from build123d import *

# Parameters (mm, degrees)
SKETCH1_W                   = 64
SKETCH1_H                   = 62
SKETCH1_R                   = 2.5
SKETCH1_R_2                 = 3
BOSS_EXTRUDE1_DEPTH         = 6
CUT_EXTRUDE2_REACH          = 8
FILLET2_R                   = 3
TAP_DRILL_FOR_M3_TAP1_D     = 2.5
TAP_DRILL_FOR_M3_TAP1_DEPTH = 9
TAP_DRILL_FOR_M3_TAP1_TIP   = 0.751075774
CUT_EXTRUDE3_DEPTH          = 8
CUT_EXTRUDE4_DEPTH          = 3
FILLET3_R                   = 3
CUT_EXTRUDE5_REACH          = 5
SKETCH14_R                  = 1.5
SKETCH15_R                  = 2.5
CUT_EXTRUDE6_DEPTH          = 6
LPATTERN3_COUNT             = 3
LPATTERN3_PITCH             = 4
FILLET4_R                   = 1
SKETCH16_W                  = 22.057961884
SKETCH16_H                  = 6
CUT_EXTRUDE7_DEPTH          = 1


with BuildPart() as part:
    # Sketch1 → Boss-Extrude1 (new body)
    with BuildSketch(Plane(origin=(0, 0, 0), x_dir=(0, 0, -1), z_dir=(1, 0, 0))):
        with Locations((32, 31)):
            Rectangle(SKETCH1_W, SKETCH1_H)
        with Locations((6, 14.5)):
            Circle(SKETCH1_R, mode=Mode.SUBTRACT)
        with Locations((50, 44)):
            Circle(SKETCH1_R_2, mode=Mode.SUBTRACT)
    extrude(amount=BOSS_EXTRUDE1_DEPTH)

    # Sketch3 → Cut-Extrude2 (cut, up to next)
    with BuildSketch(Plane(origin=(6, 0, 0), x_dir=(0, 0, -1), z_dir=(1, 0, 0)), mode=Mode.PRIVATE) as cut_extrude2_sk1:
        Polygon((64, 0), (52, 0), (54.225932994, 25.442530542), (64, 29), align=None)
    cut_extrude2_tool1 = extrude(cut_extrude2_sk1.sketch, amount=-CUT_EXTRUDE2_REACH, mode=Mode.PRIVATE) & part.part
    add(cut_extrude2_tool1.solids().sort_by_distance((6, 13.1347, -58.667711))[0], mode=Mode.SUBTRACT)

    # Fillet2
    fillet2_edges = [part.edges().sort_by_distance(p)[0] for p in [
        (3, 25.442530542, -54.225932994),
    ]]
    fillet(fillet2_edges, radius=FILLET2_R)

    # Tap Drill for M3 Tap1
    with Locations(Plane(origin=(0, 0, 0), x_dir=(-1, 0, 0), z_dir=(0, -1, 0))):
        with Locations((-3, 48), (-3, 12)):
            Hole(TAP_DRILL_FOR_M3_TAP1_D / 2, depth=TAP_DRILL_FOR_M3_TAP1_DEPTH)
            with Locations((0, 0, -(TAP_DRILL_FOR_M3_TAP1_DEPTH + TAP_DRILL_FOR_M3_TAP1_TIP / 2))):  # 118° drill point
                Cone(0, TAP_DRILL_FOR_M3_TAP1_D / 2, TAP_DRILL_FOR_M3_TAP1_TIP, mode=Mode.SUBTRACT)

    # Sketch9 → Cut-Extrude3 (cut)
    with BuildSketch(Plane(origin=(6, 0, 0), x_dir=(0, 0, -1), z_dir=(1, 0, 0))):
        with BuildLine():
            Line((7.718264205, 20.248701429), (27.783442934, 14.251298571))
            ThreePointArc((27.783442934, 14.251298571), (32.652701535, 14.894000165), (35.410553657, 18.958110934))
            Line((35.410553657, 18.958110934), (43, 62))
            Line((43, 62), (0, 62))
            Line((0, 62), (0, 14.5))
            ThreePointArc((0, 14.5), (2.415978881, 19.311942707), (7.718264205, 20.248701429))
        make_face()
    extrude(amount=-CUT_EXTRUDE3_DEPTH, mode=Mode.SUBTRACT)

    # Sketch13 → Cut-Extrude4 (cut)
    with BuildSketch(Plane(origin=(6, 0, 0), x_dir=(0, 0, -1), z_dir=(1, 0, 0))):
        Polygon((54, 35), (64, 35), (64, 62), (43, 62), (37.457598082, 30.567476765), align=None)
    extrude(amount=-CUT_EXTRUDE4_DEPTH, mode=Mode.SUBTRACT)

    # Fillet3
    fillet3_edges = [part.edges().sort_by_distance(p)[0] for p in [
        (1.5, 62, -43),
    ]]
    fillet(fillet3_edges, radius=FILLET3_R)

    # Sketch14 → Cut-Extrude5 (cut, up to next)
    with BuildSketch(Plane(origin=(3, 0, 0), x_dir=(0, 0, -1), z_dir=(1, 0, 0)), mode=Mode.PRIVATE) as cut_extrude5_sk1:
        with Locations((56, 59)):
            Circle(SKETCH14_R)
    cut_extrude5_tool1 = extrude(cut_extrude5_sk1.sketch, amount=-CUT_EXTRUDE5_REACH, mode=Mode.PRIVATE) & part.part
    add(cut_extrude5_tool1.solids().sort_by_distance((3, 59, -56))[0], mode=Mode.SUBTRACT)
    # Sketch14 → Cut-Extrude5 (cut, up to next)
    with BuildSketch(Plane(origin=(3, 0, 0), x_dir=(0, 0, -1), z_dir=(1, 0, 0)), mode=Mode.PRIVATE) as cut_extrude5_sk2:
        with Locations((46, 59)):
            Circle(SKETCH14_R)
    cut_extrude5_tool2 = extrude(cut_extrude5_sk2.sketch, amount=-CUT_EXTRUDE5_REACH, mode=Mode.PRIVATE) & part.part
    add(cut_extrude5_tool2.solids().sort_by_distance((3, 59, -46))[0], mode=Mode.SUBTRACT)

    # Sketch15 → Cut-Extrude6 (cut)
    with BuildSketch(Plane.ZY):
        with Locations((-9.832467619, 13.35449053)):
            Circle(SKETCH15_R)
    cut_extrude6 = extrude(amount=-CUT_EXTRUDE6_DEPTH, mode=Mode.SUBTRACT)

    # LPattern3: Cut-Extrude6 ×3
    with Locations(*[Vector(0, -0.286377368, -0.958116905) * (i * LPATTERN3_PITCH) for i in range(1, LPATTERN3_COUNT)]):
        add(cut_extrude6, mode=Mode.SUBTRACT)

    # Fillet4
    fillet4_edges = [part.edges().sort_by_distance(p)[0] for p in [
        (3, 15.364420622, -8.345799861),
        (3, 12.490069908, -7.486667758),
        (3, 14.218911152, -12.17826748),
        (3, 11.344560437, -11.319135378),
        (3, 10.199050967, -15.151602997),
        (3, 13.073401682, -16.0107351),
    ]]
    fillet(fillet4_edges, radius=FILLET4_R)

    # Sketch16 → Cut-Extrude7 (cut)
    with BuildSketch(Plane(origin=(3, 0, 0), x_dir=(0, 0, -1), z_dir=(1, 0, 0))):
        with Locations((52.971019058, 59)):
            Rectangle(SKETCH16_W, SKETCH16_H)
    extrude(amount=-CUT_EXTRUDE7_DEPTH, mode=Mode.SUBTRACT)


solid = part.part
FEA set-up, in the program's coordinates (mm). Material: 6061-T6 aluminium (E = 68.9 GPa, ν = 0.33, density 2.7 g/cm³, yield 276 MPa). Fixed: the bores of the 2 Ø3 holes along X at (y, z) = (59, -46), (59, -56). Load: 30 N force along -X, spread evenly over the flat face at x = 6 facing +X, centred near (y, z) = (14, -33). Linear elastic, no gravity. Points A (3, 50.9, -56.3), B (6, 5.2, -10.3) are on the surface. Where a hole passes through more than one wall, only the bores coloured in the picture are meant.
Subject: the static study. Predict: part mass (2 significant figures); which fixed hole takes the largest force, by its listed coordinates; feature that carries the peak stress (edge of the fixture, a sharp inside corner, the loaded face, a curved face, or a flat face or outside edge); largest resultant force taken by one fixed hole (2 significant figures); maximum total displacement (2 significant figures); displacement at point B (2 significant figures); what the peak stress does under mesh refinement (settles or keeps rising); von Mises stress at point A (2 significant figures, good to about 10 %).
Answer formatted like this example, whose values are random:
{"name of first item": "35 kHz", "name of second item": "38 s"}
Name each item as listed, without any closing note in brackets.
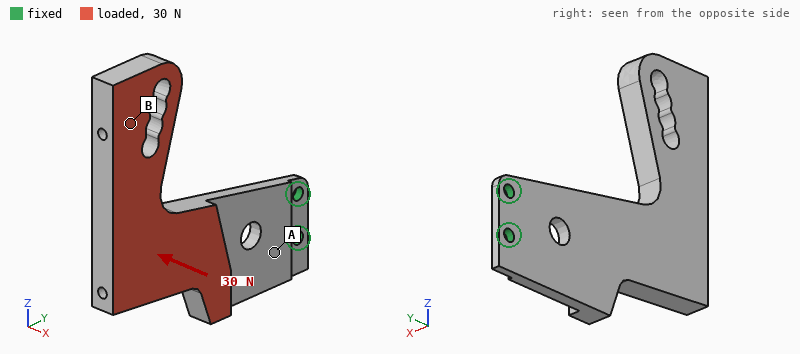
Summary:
{"part mass": "24 g", "which fixed hole takes the largest force, by its listed coordinates": "(59, -46)", "feature that carries the peak stress": "edge of the fixture", "largest resultant force taken by one fixed hole": "50 N", "maximum total displacement": "0.66 mm", "displacement at point B": "0.58 mm", "what the peak stress does under mesh refinement": "keeps rising", "von Mises stress at point A": "32 MPa"}
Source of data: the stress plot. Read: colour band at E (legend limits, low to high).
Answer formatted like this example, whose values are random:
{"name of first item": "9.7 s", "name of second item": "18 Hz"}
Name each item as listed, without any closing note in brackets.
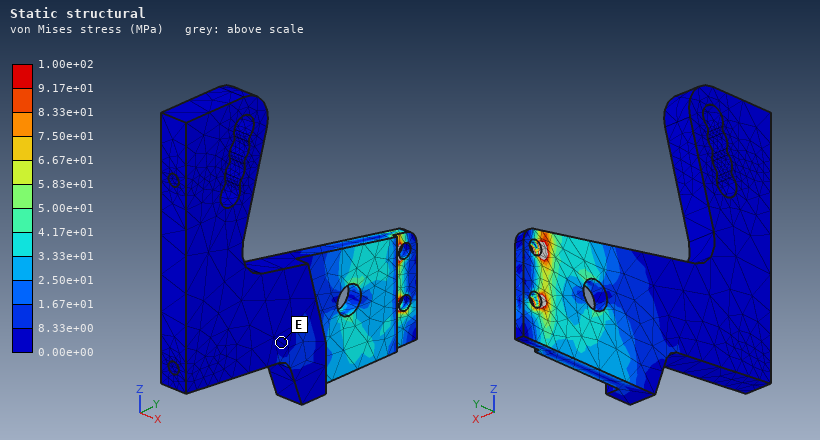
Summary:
{"colour band at E": "0.00e+00 to 8.33e+00 MPa"}
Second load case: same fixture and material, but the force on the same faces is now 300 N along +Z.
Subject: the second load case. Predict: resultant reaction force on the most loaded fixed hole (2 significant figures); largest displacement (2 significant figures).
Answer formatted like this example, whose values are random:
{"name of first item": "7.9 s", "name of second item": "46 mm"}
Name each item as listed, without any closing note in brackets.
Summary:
{"resultant reaction force on the most loaded fixed hole": "1.1 kN", "largest displacement": "0.32 mm"}
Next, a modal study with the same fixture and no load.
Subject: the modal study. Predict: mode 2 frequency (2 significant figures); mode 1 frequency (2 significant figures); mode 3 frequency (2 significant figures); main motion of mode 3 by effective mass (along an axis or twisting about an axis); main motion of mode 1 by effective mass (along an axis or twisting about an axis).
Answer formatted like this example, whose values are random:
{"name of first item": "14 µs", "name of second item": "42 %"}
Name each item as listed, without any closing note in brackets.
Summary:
{"mode 2 frequency": "1100 Hz", "mode 1 frequency": "290 Hz", "mode 3 frequency": "1700 Hz", "main motion of mode 3 by effective mass": "along Z", "main motion of mode 1 by effective mass": "along X"}
